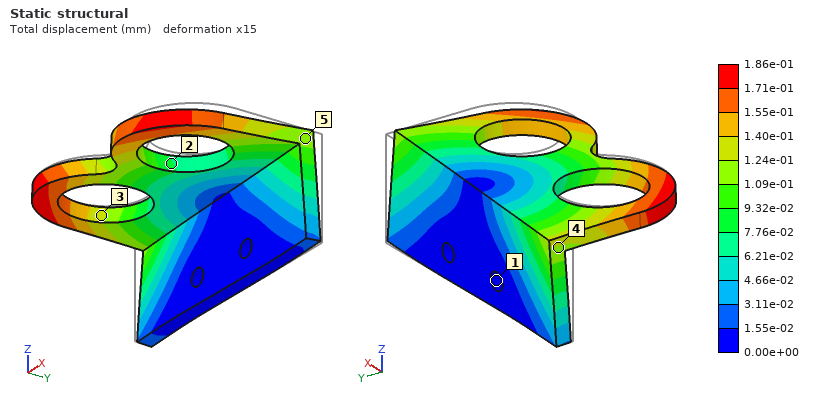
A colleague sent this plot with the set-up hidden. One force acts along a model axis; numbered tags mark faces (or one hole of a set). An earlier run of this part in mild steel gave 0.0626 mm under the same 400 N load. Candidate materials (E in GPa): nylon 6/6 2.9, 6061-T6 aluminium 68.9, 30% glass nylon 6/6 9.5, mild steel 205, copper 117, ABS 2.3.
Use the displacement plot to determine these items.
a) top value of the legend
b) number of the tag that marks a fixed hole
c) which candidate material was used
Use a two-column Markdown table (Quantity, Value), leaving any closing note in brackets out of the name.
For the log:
| Quantity | Value |
|---|---|
| top value of the legend | 1.86e-01 mm |
| number of the tag that marks a fixed hole | 1 |
| which candidate material was used | 6061-T6 aluminium |
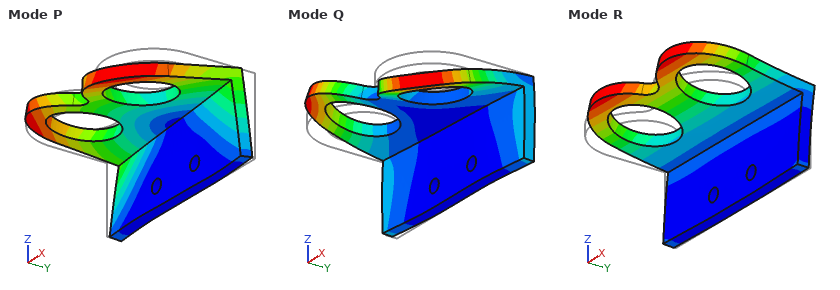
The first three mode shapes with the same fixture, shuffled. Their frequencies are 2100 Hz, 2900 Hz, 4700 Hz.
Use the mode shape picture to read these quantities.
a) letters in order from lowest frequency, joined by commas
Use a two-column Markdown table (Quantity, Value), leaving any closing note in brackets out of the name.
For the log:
| Quantity | Value |
|---|---|
| letters in order from lowest frequency, joined by commas | R, P, Q |
